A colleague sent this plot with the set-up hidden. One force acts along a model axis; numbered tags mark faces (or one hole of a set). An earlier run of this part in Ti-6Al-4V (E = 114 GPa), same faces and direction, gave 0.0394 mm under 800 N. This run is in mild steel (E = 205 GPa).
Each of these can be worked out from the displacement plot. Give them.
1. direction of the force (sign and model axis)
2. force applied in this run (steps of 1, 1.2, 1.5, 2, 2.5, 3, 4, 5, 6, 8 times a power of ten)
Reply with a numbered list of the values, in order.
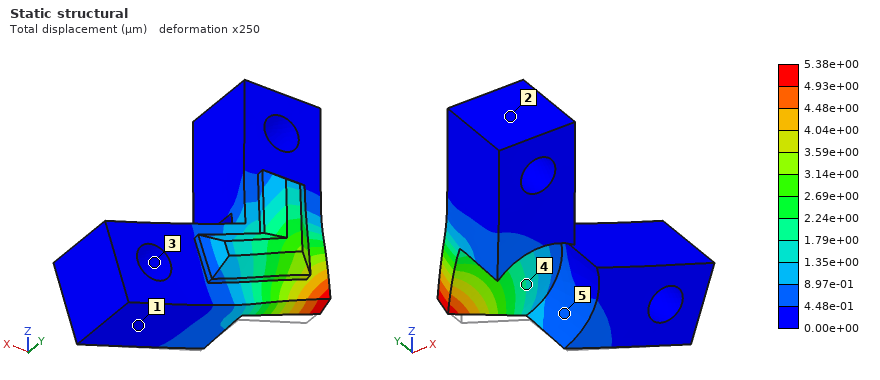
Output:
1. +Y
2. 200 N
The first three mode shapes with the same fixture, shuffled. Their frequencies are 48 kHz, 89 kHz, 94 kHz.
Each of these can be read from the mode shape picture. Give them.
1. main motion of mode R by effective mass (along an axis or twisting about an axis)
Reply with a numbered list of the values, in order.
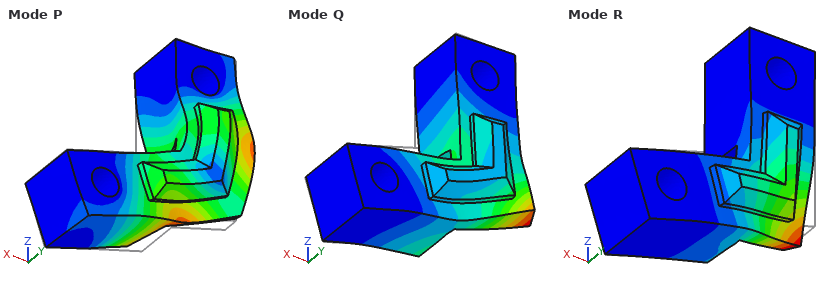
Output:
1. along Y
